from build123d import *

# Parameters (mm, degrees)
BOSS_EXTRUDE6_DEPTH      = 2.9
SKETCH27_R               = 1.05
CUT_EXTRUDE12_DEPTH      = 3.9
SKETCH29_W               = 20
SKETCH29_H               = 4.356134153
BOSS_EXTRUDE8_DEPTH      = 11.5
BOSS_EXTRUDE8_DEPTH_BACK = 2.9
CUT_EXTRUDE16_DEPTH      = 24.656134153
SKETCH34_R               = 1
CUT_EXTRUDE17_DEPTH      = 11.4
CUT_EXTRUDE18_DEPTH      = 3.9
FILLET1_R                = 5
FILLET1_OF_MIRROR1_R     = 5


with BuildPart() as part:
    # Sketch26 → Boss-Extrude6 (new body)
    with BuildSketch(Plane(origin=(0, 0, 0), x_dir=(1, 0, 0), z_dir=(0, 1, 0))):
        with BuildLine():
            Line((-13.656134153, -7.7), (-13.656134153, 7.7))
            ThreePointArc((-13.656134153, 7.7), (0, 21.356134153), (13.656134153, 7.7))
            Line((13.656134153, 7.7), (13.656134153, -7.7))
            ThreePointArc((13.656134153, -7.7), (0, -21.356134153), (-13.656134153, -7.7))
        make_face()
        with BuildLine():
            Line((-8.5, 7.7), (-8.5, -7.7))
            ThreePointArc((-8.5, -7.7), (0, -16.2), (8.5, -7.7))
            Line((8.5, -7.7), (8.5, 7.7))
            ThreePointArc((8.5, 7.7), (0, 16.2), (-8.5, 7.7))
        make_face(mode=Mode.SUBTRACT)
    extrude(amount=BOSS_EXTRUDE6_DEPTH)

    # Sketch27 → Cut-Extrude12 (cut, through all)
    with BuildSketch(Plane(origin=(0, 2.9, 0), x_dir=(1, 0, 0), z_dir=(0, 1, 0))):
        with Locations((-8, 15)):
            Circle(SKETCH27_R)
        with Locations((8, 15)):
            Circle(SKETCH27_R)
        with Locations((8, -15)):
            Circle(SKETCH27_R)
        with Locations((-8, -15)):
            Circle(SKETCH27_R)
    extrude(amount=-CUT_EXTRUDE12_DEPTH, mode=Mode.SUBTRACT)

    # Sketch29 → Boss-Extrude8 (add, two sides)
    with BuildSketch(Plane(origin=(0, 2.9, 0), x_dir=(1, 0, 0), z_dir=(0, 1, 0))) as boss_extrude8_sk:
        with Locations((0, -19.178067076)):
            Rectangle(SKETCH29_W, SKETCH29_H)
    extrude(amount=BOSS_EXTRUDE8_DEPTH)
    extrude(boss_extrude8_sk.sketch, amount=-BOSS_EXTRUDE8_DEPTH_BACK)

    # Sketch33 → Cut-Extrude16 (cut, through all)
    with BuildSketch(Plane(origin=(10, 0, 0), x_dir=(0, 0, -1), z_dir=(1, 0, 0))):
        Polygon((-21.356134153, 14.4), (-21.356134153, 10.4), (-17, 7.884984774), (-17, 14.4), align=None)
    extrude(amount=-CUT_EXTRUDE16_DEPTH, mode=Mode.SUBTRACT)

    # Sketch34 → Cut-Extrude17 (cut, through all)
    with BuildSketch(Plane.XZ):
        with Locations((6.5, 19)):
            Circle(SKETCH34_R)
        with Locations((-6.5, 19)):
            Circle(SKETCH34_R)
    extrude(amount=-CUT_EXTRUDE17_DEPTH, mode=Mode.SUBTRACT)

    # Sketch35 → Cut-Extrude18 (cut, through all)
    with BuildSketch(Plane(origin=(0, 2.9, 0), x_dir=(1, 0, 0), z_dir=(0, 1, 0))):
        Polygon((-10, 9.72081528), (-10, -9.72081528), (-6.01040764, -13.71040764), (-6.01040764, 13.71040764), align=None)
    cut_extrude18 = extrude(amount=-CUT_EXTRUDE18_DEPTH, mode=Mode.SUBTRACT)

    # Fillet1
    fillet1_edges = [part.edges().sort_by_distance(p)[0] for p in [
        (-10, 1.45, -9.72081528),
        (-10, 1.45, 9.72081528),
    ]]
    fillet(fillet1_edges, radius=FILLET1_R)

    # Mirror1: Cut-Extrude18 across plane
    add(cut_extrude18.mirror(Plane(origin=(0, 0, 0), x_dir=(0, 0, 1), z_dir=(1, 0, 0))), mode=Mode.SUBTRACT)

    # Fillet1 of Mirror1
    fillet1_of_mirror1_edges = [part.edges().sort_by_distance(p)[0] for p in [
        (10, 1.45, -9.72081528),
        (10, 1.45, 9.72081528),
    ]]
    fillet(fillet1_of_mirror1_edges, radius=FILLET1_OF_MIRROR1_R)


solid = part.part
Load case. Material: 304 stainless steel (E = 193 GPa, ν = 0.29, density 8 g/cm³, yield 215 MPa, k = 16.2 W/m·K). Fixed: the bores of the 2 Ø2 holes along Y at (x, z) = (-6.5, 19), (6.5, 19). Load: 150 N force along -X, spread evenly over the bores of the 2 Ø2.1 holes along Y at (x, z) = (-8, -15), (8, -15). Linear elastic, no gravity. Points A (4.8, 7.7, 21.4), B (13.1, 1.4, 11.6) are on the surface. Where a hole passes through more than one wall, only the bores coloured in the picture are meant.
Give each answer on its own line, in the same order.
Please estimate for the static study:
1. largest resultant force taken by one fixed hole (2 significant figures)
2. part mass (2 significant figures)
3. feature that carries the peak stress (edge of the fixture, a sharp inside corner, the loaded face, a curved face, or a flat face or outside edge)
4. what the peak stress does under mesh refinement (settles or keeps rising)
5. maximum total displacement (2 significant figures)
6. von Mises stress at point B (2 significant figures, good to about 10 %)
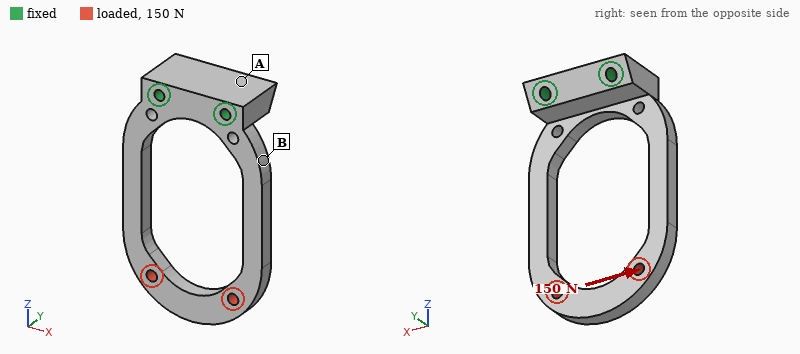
280 N
15 g
a sharp inside corner
keeps rising
87 µm
100 MPa
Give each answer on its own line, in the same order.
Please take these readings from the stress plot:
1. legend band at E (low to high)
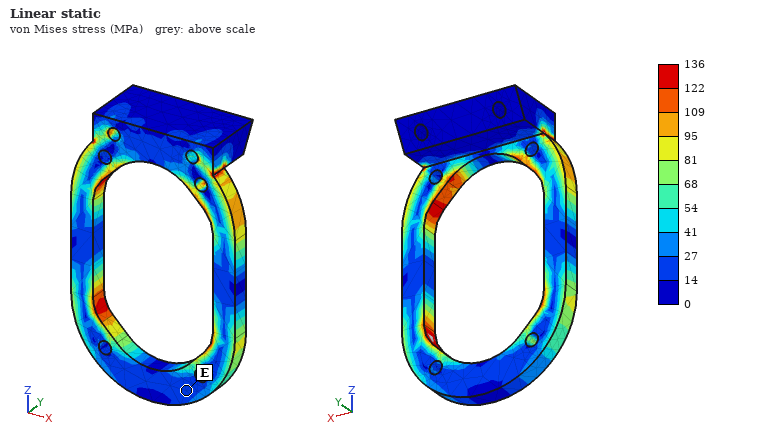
14 to 27 MPa
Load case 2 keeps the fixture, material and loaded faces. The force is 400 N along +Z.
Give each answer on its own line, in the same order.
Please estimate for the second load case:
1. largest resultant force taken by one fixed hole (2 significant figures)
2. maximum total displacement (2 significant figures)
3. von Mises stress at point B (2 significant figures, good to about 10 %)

210 N
12 µm
18 MPa
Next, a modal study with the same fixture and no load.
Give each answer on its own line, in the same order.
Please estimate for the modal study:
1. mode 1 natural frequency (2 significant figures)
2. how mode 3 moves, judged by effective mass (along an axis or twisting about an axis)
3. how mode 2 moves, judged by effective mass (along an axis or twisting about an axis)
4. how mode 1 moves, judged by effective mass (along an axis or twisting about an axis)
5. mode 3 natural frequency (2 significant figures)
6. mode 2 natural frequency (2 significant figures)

1200 Hz
twisting about Z
along X
along Y
3400 Hz
3100 Hz
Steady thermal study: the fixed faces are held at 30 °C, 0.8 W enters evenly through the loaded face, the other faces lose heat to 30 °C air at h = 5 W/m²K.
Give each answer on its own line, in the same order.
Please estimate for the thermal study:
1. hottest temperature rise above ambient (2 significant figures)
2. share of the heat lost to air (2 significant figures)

61 K
28 %
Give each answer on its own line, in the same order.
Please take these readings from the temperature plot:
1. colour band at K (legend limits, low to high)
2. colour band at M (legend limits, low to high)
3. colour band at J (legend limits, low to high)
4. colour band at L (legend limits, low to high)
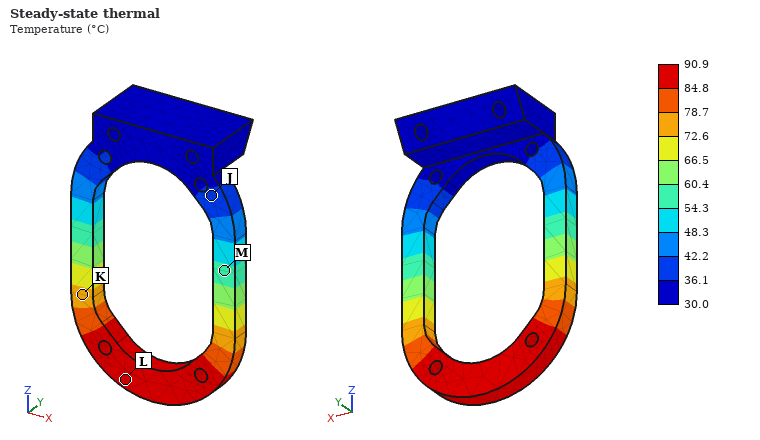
72.6 to 78.7 °C
54.3 to 60.4 °C
36.1 to 42.2 °C
84.8 to 90.9 °C
